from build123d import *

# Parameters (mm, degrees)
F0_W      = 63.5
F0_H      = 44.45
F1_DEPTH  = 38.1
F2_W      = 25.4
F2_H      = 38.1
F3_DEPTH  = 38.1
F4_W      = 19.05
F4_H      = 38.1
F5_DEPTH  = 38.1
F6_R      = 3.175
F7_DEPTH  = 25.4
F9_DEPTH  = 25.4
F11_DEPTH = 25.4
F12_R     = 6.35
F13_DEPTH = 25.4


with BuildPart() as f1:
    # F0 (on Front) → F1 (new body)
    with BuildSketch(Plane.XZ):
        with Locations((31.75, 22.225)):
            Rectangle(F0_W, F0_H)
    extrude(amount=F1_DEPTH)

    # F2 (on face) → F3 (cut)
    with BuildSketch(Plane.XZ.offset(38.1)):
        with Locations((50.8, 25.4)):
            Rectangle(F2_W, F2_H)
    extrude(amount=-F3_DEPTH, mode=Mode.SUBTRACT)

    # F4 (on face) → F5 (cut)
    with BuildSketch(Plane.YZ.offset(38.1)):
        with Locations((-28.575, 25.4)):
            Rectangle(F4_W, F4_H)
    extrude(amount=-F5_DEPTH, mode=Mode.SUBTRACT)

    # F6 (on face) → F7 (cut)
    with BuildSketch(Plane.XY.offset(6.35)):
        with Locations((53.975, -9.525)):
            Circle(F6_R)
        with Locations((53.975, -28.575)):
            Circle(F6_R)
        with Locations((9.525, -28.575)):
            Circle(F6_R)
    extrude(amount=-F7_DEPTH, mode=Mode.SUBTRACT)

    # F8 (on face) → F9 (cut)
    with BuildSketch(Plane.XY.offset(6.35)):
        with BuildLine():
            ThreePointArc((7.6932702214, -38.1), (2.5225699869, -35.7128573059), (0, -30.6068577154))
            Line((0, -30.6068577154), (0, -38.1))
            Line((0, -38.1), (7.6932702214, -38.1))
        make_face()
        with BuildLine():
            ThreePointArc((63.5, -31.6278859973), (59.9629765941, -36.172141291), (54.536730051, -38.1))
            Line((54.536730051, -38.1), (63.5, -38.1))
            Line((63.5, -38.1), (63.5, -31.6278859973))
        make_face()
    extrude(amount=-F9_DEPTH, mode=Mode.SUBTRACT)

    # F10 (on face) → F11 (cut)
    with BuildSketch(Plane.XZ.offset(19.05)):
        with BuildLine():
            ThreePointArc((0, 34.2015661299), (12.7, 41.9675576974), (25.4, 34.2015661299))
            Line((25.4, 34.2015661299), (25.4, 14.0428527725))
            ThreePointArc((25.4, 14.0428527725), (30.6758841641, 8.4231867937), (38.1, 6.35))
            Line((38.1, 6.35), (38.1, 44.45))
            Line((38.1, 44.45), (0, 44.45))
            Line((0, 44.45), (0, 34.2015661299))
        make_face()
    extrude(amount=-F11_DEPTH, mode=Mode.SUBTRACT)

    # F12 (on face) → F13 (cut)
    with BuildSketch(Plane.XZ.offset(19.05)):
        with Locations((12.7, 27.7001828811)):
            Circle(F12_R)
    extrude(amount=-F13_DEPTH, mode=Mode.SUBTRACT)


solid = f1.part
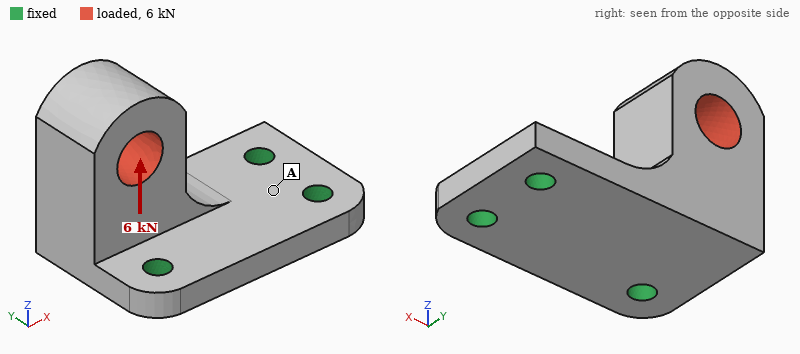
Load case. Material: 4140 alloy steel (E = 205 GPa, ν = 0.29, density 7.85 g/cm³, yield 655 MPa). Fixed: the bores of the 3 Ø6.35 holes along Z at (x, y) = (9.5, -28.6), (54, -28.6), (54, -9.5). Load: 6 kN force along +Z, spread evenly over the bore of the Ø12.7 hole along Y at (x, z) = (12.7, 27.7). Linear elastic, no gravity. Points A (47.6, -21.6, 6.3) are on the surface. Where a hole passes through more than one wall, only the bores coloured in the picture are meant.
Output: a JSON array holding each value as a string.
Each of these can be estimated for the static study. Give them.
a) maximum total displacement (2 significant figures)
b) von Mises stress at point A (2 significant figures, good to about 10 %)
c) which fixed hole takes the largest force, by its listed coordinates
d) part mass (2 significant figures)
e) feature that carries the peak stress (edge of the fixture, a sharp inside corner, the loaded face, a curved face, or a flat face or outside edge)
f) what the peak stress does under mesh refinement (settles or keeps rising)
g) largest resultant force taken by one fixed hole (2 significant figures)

["0.16 mm", "62 MPa", "(9.5, -28.6)", "230 g", "edge of the fixture", "keeps rising", "4.9 kN"]
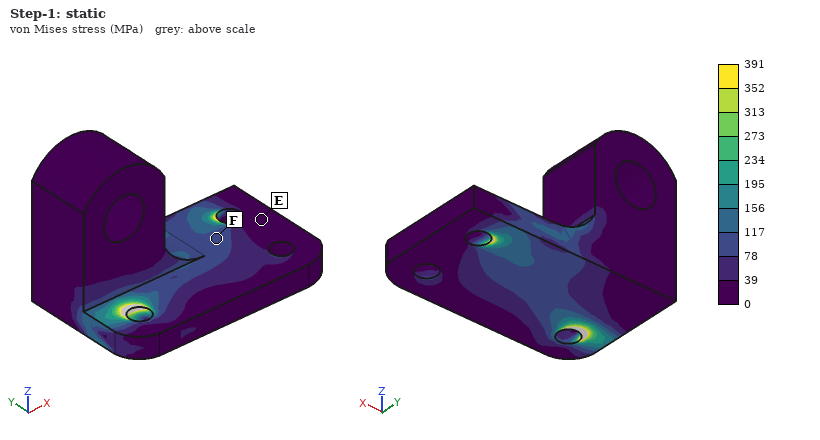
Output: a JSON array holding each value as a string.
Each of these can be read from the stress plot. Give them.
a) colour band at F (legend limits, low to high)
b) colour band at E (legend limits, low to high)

["78 to 117 MPa", "0 to 39 MPa"]
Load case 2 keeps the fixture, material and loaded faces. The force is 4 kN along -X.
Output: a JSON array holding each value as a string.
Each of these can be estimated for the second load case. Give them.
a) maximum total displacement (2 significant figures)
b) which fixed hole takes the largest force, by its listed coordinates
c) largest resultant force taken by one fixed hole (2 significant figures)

["77 µm", "(9.5, -28.6)", "2.7 kN"]
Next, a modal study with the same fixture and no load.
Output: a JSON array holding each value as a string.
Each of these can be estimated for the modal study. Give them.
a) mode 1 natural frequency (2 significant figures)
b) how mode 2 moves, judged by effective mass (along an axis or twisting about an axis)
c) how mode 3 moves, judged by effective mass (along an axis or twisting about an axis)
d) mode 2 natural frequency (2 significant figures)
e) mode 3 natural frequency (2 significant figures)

["2600 Hz", "along X", "along Z", "5500 Hz", "9600 Hz"]
